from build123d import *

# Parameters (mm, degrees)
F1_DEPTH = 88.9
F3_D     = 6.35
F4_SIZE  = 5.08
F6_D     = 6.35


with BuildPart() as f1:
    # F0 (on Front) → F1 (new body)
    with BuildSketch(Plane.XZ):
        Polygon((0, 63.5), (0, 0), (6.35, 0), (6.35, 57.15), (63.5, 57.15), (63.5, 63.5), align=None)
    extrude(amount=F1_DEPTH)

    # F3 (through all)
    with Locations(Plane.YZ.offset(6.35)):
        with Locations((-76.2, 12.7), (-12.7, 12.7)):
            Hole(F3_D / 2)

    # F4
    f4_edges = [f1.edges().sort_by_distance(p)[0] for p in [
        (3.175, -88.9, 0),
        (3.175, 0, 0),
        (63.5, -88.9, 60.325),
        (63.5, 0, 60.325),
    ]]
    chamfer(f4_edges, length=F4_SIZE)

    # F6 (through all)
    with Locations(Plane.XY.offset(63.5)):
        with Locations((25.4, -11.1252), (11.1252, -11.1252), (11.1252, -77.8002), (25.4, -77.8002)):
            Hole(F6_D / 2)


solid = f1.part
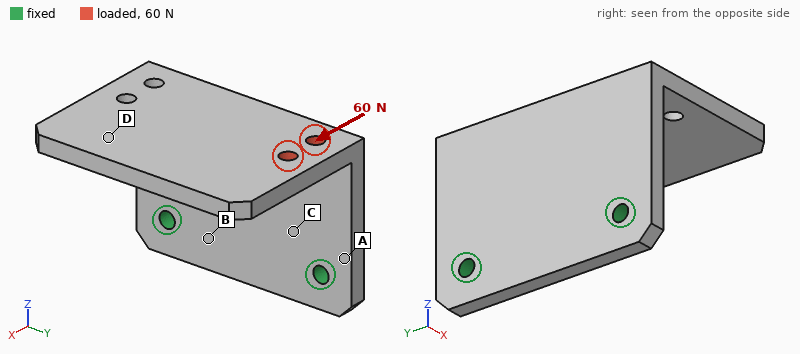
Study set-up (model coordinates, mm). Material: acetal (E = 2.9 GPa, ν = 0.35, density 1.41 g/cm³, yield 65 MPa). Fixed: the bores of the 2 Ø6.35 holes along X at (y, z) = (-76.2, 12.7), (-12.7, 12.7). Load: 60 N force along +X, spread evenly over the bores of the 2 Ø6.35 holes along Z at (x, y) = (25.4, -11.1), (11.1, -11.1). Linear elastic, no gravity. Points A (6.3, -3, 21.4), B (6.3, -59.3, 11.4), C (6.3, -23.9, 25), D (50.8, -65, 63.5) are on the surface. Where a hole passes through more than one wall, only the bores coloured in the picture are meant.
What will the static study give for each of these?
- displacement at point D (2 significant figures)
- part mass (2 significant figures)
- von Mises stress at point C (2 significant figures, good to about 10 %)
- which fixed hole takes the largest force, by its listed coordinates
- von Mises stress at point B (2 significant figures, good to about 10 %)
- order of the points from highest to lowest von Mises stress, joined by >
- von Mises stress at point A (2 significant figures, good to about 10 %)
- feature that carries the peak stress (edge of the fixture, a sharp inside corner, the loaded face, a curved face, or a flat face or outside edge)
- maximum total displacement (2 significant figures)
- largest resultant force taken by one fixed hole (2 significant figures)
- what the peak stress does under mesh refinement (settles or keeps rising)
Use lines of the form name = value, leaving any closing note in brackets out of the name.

displacement at point D = 0.75 mm
part mass = 94 g
von Mises stress at point C = 4.1 MPa
which fixed hole takes the largest force, by its listed coordinates = (-12.7, 12.7)
von Mises stress at point B = 1.9 MPa
order of the points from highest to lowest von Mises stress, joined by > = A > C > B > D
von Mises stress at point A = 6.6 MPa
feature that carries the peak stress = edge of the fixture
maximum total displacement = 1.2 mm
largest resultant force taken by one fixed hole = 60 N
what the peak stress does under mesh refinement = keeps rising
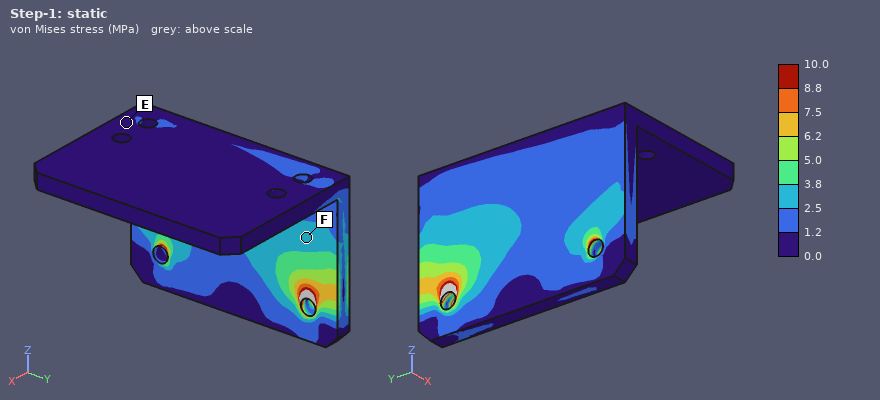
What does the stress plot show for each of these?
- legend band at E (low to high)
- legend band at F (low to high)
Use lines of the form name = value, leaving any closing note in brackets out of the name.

legend band at E = 0.0 to 1.2 MPa
legend band at F = 2.5 to 3.8 MPa
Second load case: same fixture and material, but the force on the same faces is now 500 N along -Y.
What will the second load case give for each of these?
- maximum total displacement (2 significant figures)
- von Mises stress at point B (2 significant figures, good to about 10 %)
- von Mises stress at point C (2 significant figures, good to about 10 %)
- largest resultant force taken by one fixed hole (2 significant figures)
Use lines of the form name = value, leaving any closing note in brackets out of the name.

maximum total displacement = 1.5 mm
von Mises stress at point B = 2.2 MPa
von Mises stress at point C = 7.0 MPa
largest resultant force taken by one fixed hole = 450 N
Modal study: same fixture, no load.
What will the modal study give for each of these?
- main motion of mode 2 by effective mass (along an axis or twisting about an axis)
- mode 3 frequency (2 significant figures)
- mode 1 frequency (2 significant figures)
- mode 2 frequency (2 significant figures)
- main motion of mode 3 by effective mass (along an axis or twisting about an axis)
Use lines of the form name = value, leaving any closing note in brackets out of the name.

main motion of mode 2 by effective mass = along Y
mode 3 frequency = 450 Hz
mode 1 frequency = 160 Hz
mode 2 frequency = 320 Hz
main motion of mode 3 by effective mass = along X
